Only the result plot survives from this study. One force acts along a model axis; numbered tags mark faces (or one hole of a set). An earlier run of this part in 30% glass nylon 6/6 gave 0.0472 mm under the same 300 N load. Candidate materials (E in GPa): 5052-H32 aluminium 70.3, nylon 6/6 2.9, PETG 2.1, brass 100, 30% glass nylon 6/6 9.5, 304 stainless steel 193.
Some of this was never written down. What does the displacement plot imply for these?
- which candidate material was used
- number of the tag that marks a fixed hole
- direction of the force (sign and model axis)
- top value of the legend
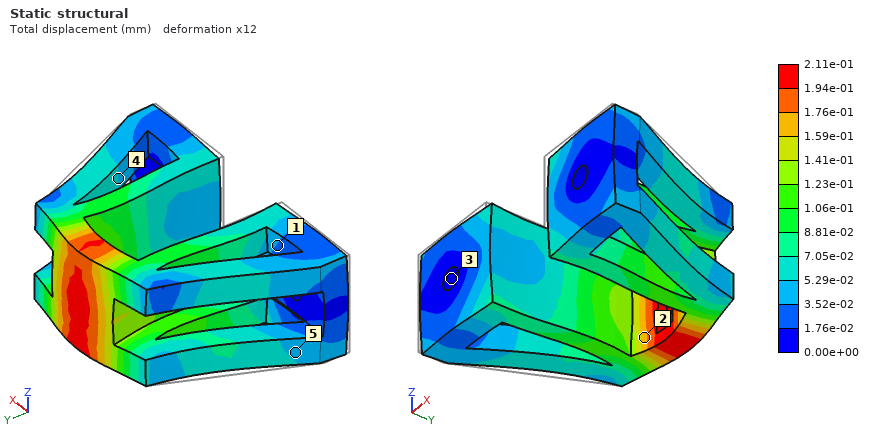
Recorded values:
PETG
3
+Y
2.11e-01 mm
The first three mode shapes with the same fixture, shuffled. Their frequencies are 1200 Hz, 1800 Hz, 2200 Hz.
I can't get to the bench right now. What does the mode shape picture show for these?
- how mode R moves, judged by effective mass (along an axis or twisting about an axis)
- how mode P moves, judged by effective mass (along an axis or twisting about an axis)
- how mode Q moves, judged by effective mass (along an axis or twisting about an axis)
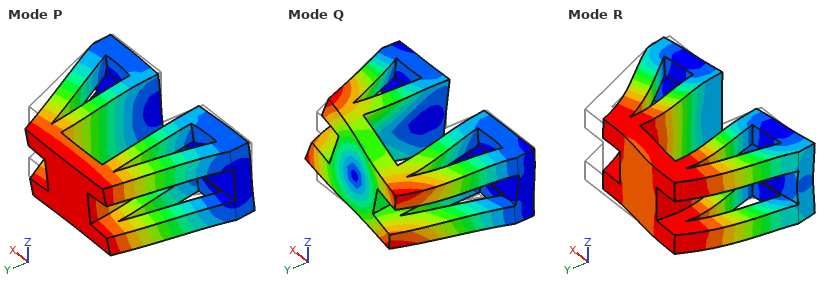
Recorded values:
along X
along Z
twisting about Y
